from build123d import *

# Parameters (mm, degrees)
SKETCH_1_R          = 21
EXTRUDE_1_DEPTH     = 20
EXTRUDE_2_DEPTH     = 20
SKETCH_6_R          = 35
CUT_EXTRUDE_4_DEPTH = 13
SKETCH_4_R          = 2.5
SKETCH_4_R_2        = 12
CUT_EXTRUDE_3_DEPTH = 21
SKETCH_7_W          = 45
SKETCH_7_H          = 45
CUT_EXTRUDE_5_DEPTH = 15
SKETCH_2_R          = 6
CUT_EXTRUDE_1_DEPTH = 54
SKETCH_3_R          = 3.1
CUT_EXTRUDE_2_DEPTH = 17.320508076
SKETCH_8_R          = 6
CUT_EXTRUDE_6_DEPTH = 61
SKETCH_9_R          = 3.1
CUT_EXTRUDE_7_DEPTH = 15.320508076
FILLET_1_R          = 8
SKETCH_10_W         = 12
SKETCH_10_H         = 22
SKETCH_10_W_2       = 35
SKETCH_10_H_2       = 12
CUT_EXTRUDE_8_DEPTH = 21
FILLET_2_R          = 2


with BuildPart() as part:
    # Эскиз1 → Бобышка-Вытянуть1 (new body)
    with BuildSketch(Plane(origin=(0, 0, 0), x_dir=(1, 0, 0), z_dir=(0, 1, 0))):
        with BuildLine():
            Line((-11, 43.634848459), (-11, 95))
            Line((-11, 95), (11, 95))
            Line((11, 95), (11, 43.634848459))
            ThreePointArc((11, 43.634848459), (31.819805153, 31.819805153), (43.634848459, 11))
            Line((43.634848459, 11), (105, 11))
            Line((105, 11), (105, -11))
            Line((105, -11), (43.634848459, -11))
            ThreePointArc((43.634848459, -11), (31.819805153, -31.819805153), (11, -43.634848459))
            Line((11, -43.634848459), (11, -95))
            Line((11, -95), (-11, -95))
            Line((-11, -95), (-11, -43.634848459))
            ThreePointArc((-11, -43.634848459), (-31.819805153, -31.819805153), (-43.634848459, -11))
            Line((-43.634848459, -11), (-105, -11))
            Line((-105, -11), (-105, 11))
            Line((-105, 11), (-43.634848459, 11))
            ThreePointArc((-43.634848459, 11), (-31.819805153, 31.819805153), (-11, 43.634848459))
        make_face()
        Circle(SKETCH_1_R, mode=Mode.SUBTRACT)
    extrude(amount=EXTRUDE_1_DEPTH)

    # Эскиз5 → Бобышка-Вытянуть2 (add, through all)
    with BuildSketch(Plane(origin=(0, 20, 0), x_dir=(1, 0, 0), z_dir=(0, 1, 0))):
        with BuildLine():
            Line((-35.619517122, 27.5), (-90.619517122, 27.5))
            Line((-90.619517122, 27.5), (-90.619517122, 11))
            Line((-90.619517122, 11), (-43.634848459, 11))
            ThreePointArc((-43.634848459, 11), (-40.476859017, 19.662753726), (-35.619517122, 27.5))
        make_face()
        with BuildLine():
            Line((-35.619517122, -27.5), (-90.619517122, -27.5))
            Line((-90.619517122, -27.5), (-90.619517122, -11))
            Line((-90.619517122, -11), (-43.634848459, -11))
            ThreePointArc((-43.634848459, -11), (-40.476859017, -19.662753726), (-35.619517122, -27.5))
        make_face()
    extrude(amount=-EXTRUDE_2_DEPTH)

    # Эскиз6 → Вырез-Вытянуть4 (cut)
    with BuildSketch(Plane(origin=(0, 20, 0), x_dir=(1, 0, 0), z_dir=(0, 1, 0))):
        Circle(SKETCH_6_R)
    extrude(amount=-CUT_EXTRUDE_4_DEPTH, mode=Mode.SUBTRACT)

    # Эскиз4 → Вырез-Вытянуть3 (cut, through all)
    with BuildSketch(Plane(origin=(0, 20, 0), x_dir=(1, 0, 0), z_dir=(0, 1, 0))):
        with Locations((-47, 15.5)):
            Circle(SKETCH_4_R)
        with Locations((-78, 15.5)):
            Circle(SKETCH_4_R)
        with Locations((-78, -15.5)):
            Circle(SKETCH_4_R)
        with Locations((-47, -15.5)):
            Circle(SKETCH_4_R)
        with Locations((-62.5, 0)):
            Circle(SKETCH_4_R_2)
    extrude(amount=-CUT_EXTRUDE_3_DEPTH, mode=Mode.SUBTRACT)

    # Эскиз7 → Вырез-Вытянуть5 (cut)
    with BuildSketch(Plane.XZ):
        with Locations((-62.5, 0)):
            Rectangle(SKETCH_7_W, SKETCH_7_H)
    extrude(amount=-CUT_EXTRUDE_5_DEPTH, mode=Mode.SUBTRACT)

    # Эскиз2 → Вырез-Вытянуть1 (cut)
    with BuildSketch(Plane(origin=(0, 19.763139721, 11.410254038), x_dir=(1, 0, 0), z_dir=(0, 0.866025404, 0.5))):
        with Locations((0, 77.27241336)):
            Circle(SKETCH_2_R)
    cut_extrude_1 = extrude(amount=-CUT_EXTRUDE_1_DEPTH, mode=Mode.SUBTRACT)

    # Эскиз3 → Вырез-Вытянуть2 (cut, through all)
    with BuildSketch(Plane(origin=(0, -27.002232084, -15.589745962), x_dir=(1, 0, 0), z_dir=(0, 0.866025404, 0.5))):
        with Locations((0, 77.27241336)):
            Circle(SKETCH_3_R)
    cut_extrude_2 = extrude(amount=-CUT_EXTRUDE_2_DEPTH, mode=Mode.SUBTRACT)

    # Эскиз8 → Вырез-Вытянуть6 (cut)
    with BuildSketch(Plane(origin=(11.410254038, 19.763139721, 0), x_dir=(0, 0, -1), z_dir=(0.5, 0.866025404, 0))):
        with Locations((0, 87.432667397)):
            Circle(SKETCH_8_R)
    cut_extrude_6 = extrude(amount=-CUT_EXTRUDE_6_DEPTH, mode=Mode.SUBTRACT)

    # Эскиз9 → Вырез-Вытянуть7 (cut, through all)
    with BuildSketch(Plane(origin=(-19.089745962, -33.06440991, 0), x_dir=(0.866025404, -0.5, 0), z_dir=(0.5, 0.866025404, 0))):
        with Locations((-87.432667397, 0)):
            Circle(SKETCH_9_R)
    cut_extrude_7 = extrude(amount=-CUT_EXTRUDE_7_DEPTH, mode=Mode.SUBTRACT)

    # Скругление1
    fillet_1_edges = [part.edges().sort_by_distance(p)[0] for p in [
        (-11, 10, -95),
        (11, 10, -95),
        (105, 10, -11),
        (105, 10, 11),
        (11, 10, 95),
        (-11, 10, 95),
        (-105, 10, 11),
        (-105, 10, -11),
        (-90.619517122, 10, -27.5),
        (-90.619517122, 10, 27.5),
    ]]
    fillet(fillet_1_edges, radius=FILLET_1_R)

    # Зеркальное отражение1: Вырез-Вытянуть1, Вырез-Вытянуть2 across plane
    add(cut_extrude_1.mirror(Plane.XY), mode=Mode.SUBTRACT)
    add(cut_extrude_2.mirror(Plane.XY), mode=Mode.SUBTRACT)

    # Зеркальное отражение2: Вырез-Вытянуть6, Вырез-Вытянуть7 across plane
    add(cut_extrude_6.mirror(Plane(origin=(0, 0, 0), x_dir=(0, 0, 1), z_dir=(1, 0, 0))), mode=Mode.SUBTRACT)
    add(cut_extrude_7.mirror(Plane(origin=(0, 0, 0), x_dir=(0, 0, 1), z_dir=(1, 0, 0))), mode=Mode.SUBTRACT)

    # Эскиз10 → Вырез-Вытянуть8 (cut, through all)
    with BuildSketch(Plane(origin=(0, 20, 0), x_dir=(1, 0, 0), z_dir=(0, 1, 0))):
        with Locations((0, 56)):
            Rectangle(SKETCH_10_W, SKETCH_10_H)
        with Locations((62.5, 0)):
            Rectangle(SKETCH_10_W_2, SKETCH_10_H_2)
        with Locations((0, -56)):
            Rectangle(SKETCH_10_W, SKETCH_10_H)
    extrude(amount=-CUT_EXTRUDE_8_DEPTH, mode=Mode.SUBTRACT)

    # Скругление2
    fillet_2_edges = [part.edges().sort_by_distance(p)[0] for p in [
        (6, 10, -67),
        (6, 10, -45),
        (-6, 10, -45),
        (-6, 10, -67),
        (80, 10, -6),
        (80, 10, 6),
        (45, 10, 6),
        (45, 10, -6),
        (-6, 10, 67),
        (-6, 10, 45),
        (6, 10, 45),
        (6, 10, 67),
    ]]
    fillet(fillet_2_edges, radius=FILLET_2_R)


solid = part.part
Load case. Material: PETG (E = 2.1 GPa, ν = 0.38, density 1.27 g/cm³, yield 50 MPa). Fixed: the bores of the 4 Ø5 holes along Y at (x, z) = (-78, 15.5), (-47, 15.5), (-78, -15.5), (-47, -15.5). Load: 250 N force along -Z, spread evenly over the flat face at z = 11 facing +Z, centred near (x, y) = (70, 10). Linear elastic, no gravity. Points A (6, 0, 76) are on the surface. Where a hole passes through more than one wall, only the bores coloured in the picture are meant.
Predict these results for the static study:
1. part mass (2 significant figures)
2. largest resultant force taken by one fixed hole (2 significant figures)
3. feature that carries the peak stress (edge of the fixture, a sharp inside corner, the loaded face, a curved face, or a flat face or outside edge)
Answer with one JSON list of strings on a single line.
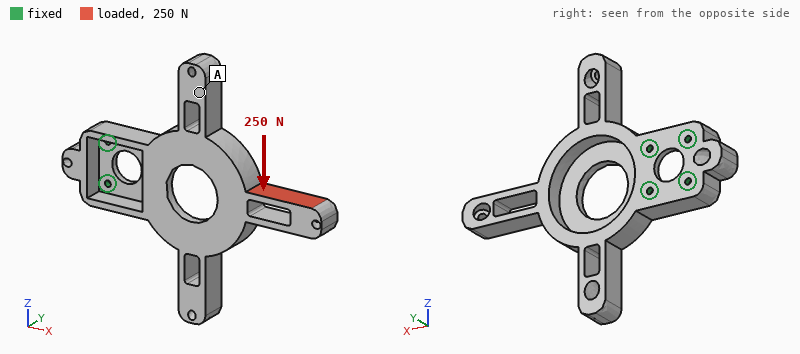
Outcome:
["170 g", "450 N", "a curved face"]
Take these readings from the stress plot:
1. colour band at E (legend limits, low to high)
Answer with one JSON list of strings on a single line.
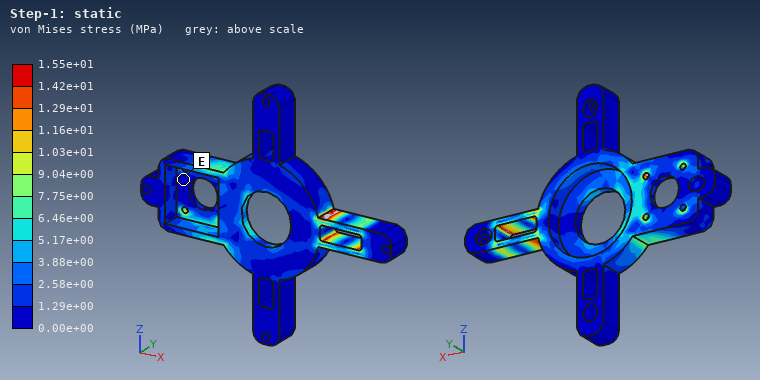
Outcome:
["0.00e+00 to 1.29e+00 MPa"]
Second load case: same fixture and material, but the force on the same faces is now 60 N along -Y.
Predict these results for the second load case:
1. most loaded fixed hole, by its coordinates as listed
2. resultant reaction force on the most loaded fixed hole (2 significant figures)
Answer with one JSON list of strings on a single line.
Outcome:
["(-47, 15.5)", "180 N"]
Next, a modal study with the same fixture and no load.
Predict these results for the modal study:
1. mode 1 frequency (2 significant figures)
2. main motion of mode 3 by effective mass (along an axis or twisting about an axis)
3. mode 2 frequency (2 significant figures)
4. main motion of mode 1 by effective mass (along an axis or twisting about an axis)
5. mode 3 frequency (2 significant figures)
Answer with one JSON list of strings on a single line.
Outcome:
["140 Hz", "along Z", "220 Hz", "along Y", "330 Hz"]
